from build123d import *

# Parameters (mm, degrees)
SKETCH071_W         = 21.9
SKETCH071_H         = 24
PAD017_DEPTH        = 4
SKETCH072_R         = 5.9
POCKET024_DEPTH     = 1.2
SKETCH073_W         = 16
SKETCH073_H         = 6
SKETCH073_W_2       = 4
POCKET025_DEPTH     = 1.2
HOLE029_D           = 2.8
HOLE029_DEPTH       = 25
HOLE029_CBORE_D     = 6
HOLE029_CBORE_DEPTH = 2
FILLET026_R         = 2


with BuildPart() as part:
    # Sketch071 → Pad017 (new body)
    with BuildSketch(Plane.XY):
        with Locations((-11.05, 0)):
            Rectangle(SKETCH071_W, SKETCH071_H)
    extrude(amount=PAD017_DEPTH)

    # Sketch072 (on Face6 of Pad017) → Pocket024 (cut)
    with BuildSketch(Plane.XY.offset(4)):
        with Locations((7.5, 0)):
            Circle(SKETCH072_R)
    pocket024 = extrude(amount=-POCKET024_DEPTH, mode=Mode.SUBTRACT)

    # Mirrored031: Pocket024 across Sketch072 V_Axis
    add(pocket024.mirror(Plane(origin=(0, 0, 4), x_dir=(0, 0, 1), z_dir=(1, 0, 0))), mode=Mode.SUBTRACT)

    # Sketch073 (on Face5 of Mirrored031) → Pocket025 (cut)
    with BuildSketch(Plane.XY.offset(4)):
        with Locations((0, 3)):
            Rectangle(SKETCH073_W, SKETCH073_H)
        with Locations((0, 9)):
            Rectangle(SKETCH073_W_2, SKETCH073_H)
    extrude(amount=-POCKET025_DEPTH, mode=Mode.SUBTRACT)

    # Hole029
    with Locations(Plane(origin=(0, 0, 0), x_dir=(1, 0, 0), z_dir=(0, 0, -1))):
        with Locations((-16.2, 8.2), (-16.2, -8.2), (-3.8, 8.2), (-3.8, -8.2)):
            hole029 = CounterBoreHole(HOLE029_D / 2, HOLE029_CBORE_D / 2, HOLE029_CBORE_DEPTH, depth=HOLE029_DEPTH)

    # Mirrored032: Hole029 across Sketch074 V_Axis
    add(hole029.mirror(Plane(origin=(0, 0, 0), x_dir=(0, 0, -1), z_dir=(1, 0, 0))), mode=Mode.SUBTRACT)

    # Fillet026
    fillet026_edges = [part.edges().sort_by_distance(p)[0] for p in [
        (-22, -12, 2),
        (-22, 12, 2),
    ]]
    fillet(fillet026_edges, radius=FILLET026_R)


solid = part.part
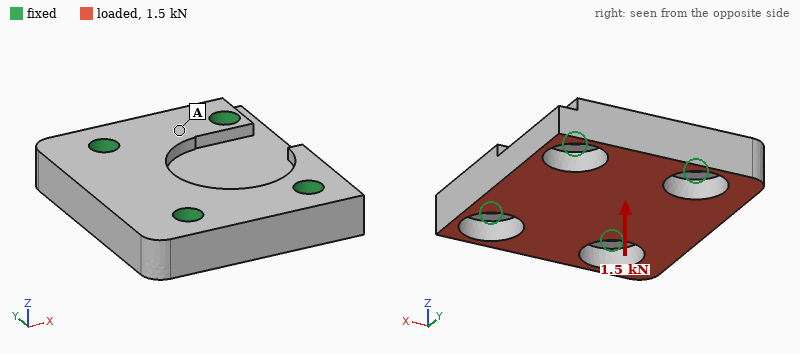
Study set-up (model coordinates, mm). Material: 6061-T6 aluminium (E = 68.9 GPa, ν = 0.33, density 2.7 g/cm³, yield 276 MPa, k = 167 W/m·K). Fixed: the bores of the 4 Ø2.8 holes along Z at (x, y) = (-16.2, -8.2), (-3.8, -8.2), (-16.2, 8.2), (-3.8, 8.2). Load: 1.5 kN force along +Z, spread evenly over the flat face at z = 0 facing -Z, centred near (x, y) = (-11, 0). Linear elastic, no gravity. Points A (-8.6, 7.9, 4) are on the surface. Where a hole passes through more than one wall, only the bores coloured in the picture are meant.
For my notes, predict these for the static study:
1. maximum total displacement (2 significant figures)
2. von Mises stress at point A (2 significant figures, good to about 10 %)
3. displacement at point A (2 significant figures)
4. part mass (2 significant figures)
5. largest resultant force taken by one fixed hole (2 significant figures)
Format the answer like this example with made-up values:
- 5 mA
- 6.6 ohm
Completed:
- 8.1 µm
- 14 MPa
- 2.8 µm
- 4.5 g
- 470 N
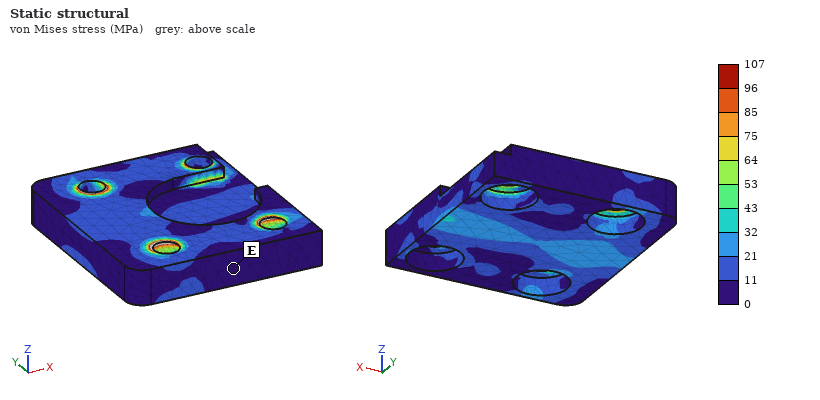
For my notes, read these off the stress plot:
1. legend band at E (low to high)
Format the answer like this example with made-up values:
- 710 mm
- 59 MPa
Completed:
- 0 to 11 MPa
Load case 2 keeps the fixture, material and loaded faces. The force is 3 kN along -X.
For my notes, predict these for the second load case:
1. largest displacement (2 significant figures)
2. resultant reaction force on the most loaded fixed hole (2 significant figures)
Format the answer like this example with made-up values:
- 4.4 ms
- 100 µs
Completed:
- 17 µm
- 890 N
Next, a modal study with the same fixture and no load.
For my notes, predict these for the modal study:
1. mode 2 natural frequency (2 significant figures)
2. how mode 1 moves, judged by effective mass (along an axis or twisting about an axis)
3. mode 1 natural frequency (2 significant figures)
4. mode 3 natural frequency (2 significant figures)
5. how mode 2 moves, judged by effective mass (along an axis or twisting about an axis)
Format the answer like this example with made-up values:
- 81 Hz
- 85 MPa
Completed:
- 44 kHz
- along Z
- 39 kHz
- 55 kHz
- along Z
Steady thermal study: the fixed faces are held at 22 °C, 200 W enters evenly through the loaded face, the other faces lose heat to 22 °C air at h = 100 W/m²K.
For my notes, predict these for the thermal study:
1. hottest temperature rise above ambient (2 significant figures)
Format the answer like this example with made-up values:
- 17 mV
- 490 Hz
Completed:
- 54 K
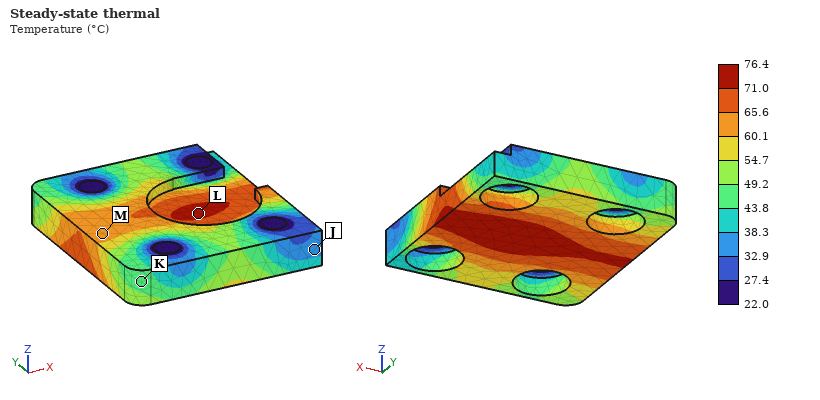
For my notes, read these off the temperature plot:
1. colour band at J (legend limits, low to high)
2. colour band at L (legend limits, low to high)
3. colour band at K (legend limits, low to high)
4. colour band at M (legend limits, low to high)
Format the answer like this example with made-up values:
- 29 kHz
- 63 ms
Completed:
- 32.9 to 38.3 °C
- 71.0 to 76.4 °C
- 43.8 to 49.2 °C
- 60.1 to 65.6 °C
